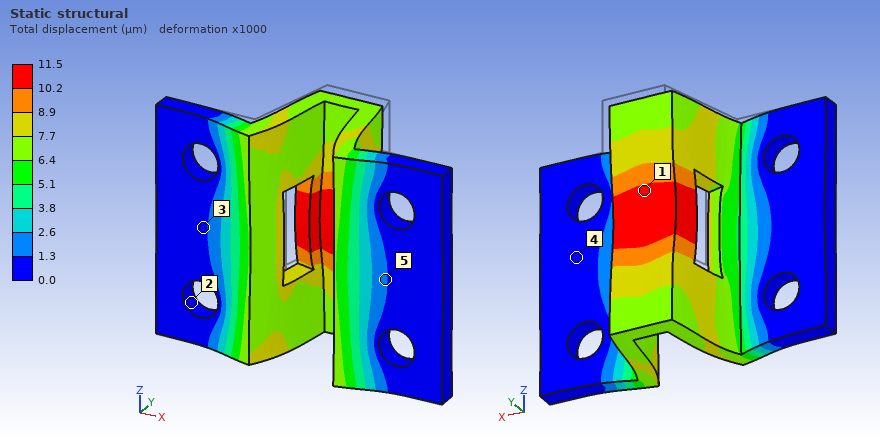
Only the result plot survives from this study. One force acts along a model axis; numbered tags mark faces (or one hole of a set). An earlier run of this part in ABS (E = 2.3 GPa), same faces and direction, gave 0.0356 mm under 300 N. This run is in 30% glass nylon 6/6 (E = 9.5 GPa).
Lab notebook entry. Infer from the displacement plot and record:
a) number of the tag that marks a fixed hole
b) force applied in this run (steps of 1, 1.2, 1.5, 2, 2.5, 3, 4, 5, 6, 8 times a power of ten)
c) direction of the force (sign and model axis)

2
400 N
-Y
